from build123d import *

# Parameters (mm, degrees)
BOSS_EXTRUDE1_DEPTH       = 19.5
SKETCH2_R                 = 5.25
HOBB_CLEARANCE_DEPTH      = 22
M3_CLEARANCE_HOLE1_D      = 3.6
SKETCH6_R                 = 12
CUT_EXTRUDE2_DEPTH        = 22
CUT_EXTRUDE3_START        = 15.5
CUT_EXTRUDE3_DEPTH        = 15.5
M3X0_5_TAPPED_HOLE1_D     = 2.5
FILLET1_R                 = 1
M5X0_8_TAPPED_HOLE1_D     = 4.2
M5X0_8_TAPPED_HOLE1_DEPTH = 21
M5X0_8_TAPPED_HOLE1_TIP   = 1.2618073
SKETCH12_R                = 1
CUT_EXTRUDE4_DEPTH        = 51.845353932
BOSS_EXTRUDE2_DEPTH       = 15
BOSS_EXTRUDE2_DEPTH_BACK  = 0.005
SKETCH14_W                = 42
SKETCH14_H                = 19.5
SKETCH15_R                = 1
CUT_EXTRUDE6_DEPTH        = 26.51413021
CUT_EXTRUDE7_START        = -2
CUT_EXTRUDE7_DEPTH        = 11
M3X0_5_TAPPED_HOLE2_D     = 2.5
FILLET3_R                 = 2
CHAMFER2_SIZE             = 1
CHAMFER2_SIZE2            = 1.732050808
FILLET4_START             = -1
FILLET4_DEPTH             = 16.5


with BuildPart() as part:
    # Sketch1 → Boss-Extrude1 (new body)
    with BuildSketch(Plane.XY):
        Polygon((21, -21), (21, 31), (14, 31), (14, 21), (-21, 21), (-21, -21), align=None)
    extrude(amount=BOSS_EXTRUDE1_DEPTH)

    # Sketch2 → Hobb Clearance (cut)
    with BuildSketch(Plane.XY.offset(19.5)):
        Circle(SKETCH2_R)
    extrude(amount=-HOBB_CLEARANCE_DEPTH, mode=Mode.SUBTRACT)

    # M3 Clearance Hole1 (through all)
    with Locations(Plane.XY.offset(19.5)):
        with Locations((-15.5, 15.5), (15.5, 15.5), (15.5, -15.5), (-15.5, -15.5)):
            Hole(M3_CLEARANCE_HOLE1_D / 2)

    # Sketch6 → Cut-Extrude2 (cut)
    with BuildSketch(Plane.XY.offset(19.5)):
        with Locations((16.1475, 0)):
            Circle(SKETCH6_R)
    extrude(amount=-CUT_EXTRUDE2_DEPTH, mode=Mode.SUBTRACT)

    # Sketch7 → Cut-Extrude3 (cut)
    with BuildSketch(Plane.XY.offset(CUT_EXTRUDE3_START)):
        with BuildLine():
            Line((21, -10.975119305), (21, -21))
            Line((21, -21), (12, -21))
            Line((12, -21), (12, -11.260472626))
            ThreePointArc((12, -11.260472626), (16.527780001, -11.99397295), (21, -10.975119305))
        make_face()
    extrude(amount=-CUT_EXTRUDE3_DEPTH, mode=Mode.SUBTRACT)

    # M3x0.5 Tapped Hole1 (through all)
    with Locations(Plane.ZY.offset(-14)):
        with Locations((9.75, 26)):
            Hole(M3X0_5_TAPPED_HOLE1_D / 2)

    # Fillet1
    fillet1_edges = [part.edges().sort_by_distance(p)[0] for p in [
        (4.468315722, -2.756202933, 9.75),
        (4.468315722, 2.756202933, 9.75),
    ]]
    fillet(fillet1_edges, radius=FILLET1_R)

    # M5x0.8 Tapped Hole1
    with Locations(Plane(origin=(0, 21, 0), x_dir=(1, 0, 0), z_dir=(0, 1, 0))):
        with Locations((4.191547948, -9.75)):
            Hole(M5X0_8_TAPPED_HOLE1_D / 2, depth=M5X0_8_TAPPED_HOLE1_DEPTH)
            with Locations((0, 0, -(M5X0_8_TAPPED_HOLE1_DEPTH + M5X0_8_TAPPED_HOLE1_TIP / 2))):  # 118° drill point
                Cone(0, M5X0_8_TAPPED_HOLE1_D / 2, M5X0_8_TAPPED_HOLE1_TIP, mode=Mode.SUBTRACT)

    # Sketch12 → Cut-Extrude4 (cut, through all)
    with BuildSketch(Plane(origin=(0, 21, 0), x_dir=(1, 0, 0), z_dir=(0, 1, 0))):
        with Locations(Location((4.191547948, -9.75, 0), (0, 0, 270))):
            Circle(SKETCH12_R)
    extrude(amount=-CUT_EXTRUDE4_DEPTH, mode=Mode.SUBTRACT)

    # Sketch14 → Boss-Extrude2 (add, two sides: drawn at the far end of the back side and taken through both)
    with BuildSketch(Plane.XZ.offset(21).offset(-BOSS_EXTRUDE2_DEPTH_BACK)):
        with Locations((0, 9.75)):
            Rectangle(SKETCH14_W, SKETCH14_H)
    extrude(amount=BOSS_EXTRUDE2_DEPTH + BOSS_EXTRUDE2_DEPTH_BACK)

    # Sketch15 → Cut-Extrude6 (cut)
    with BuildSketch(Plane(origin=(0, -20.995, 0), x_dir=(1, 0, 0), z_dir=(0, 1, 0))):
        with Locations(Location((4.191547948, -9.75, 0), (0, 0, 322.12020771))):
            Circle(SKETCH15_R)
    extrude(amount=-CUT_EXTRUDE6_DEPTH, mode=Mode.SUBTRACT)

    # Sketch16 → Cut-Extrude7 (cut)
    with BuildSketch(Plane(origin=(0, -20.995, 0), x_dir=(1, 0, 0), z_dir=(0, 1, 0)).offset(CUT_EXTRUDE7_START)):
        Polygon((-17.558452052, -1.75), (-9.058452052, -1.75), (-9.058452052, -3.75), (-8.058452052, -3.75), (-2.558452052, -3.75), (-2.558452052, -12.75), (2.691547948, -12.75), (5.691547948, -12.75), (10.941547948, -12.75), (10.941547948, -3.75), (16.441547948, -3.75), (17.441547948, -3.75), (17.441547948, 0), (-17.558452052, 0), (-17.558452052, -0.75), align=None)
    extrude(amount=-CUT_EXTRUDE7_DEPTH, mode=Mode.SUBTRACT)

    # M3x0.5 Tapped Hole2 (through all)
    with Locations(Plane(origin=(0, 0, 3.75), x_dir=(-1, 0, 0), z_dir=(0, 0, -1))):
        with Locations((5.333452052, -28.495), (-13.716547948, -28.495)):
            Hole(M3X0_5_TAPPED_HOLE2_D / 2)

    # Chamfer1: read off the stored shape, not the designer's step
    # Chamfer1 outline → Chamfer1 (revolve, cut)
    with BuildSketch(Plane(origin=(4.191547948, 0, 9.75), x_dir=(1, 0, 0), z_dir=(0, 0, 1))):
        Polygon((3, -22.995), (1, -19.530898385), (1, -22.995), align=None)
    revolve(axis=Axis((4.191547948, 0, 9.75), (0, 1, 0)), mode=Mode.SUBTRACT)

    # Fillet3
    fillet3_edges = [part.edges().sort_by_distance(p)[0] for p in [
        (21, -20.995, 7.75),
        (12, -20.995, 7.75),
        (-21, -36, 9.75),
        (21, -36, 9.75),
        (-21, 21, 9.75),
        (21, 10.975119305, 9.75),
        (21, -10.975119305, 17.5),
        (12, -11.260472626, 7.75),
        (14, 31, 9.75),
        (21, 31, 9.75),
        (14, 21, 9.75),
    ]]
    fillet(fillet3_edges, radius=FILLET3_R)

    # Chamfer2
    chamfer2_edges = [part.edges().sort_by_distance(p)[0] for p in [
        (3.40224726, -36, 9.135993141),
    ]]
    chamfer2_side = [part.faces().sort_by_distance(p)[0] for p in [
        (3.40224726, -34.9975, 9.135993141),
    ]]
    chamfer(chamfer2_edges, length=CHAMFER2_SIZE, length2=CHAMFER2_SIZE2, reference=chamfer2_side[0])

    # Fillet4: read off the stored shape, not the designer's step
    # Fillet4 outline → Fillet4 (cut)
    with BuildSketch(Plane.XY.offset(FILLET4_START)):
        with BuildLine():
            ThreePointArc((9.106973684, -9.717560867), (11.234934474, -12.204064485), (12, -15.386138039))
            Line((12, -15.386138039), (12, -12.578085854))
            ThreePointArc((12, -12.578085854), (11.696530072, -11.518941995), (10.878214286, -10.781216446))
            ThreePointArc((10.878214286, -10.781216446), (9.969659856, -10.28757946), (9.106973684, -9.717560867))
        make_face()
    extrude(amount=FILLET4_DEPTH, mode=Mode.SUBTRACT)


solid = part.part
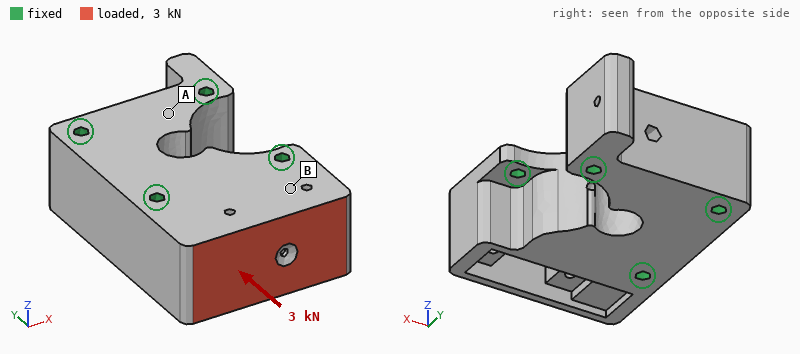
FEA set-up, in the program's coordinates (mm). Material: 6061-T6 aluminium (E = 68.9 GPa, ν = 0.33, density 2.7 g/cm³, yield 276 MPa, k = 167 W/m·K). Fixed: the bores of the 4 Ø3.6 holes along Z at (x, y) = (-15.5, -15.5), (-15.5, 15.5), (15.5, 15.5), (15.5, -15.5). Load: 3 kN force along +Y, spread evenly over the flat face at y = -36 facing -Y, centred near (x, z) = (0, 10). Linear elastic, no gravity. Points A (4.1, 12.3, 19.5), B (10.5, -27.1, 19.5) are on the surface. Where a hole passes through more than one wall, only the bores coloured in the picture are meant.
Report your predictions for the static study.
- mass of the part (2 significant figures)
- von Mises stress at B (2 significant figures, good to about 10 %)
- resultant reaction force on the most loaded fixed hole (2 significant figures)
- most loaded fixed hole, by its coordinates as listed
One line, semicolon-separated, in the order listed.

93 g; 11 MPa; 1.5 kN; (-15.5, -15.5)
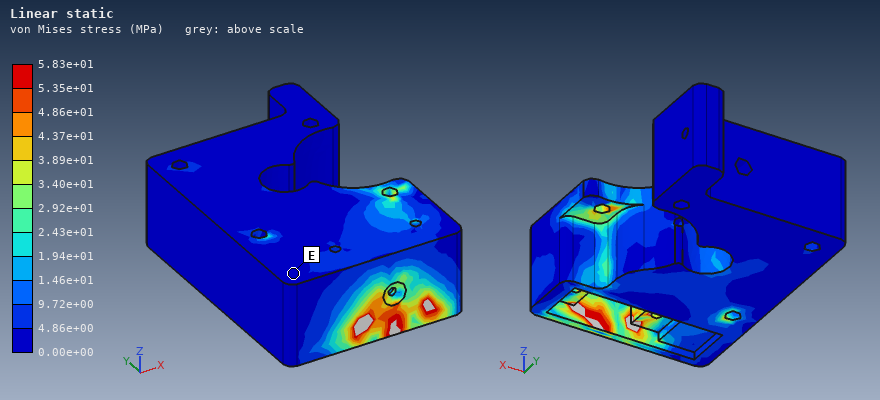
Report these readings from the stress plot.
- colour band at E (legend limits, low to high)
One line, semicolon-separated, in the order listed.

0.00e+00 to 4.86e+00 MPa
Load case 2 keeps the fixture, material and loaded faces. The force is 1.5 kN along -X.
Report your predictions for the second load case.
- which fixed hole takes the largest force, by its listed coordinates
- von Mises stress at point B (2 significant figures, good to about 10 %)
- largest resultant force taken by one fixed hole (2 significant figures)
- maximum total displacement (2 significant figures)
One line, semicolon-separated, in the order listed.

(-15.5, -15.5); 8.9 MPa; 1.6 kN; 9.9 µm
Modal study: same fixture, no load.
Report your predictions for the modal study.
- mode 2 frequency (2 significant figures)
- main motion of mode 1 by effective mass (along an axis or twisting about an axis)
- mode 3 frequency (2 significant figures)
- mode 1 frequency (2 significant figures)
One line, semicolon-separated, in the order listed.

20 kHz; along Z; 24 kHz; 13 kHz
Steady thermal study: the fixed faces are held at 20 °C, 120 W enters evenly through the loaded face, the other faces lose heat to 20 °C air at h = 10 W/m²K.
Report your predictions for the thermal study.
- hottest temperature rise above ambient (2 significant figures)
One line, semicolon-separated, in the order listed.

54 K
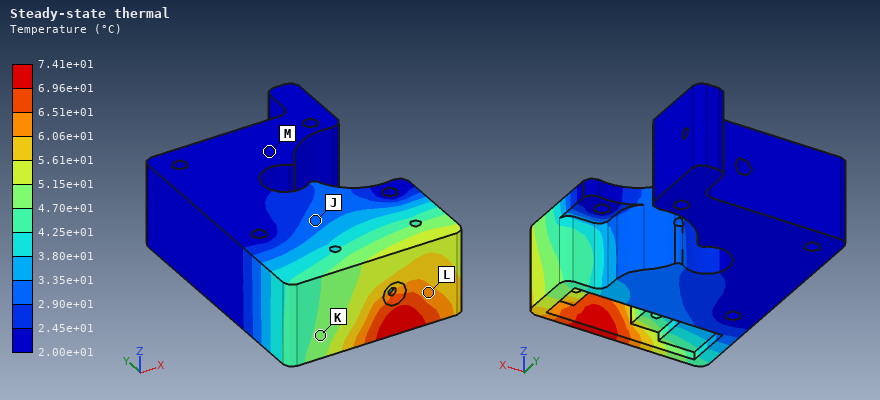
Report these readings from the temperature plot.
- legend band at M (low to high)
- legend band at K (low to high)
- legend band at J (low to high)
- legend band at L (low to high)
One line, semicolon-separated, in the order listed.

2.00e+01 to 2.45e+01 °C; 4.70e+01 to 5.15e+01 °C; 2.90e+01 to 3.35e+01 °C; 6.06e+01 to 6.51e+01 °C
